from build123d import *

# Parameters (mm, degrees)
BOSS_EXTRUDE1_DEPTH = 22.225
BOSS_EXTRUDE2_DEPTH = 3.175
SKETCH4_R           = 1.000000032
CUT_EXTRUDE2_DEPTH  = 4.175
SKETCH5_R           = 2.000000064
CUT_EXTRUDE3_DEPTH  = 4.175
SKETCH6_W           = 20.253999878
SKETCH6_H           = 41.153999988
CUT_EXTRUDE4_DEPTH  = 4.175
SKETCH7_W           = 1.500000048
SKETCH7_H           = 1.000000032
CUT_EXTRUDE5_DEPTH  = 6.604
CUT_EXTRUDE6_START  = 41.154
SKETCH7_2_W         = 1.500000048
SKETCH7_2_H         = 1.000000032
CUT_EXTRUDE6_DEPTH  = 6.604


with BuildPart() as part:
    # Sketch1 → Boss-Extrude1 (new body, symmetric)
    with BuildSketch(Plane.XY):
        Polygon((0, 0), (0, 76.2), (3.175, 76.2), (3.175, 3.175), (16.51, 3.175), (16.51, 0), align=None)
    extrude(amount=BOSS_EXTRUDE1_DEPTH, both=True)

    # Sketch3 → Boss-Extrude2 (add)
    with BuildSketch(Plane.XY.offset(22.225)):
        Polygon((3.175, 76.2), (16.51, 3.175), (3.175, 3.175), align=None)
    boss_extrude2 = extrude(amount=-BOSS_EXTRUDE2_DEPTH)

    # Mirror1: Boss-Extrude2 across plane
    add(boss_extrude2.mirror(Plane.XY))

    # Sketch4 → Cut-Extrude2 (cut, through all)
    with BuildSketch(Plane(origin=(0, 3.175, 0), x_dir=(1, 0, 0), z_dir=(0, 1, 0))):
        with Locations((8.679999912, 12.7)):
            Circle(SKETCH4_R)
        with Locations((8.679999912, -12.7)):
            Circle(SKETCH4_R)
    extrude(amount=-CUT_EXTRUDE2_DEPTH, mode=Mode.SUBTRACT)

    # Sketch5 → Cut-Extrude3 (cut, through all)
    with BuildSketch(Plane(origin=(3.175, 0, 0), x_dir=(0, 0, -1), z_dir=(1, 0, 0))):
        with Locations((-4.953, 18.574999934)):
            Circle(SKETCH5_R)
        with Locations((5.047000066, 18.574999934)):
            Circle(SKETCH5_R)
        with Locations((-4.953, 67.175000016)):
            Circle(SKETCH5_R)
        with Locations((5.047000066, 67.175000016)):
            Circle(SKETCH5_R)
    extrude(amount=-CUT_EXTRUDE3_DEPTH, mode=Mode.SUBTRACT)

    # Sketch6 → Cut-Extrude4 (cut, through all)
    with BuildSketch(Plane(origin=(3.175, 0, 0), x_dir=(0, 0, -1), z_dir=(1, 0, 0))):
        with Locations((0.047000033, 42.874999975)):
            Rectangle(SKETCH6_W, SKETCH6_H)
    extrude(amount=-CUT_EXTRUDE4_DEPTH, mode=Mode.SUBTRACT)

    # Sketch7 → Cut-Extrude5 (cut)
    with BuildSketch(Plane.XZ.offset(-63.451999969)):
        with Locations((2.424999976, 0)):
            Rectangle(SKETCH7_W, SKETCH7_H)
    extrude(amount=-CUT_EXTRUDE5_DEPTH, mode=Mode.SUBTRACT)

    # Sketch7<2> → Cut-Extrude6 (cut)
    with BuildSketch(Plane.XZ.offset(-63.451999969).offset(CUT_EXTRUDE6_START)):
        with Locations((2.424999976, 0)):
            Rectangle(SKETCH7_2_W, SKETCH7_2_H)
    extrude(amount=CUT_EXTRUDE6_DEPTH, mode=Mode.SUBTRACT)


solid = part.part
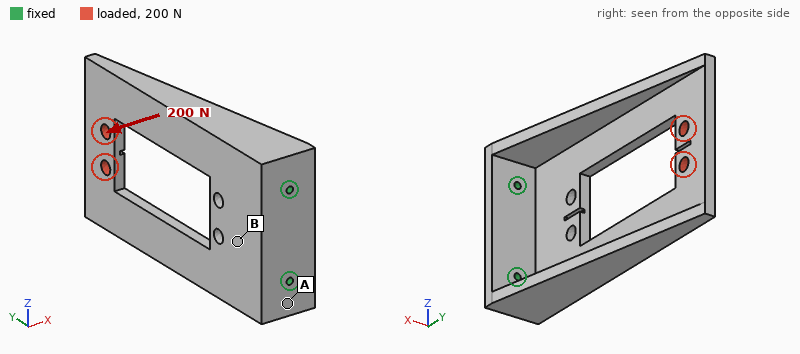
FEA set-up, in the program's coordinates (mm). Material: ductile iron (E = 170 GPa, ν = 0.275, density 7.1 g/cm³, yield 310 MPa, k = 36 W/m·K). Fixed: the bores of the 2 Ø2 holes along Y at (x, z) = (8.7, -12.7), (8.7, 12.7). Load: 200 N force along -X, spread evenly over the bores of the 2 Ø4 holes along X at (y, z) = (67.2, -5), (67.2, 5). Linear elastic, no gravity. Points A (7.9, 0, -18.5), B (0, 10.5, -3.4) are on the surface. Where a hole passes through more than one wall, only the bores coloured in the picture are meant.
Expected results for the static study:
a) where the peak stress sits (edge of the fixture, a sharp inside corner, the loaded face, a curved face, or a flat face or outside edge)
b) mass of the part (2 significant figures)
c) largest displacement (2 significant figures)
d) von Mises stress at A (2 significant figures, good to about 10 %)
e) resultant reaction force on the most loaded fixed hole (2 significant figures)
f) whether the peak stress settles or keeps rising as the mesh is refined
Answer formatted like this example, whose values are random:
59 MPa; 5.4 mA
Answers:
edge of the fixture; 91 g; 0.39 mm; 84 MPa; 110 N; keeps rising
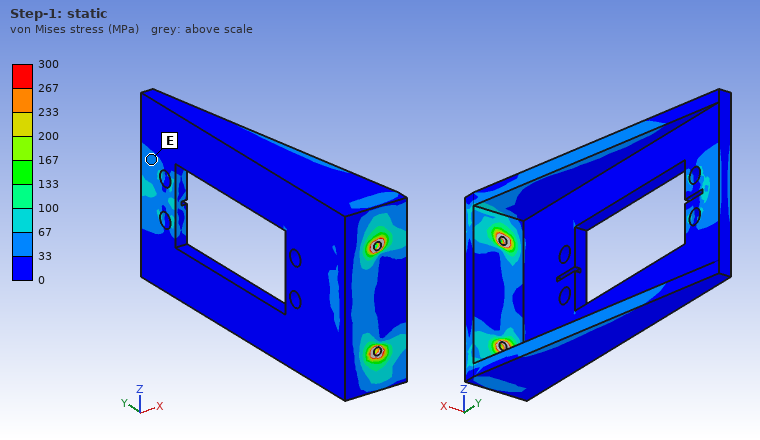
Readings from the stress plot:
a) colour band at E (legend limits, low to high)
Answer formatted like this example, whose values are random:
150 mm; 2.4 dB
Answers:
33 to 67 MPa
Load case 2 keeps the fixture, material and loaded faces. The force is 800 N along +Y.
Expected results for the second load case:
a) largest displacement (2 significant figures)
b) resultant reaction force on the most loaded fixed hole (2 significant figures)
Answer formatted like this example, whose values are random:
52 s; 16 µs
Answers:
0.11 mm; 400 N
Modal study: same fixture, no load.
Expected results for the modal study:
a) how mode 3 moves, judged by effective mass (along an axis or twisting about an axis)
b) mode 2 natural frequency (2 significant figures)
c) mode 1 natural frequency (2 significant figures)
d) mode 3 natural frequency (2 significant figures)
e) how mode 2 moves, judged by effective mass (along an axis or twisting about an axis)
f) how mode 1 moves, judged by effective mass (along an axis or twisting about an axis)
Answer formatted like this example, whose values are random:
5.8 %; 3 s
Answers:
along Z; 1400 Hz; 780 Hz; 2700 Hz; along Z; along X
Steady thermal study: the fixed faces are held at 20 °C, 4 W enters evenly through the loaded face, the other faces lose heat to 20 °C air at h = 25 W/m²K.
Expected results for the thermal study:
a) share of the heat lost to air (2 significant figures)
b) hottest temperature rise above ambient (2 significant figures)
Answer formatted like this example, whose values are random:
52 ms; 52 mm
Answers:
71 %; 46 K
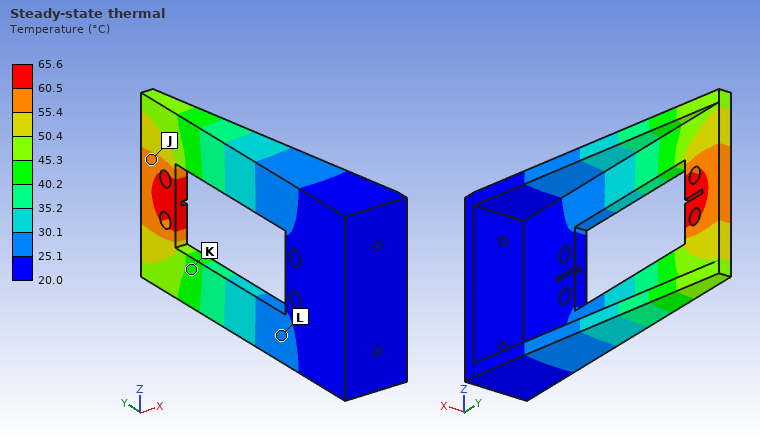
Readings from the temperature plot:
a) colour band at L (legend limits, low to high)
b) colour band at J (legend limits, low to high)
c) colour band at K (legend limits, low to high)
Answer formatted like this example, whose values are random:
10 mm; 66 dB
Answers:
25.1 to 30.1 °C; 55.4 to 60.5 °C; 40.2 to 45.3 °C
